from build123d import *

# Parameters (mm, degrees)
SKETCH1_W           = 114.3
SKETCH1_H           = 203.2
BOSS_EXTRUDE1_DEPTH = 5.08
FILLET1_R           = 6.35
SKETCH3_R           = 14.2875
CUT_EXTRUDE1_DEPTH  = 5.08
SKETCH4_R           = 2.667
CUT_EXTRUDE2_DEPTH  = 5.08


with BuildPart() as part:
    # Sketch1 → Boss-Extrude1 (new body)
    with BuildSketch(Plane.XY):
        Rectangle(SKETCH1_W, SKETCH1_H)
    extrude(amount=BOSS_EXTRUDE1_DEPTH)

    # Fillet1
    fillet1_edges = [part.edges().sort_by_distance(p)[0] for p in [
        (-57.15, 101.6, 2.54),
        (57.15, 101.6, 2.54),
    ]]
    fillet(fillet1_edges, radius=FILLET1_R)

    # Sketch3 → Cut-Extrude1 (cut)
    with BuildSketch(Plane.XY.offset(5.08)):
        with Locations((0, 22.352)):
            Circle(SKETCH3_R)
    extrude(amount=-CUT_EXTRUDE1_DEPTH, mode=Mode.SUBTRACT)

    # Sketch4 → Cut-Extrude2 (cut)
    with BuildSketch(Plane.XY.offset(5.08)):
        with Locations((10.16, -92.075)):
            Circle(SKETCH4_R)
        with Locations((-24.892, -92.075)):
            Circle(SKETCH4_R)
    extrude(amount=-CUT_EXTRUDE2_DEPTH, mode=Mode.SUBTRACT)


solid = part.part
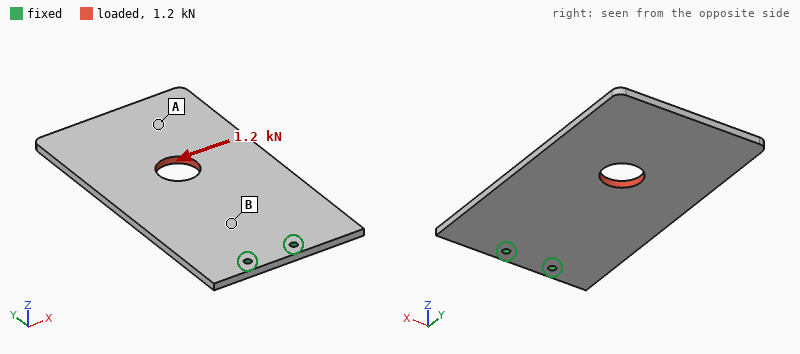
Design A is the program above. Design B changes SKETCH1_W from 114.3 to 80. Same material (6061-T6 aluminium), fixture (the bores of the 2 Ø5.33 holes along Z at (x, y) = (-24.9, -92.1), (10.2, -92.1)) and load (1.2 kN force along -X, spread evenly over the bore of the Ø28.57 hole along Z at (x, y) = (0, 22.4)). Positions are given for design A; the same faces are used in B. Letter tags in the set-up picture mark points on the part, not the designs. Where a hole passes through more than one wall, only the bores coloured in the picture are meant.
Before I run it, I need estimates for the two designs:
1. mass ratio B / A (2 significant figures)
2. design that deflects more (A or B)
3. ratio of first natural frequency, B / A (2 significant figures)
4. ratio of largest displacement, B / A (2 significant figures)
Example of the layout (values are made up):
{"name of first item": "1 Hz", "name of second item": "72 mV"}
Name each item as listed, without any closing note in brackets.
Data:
{"mass ratio B / A": "0.69", "design that deflects more": "B", "ratio of first natural frequency, B / A": "1.0", "ratio of largest displacement, B / A": "1.2"}
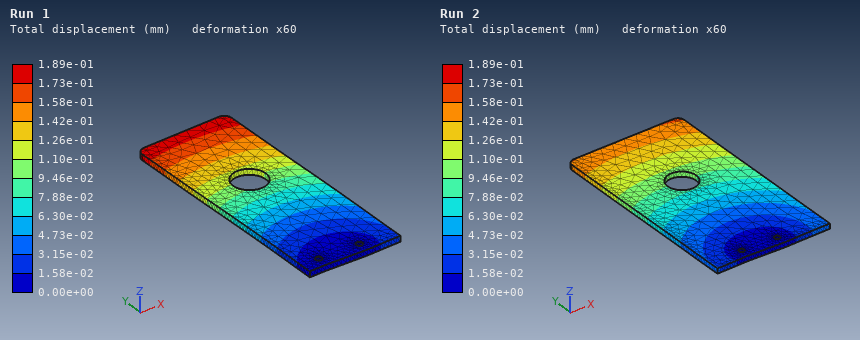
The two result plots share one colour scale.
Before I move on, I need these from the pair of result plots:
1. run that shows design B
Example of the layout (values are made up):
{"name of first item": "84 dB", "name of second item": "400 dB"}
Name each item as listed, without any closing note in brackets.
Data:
{"run that shows design B": "Run 1"}
